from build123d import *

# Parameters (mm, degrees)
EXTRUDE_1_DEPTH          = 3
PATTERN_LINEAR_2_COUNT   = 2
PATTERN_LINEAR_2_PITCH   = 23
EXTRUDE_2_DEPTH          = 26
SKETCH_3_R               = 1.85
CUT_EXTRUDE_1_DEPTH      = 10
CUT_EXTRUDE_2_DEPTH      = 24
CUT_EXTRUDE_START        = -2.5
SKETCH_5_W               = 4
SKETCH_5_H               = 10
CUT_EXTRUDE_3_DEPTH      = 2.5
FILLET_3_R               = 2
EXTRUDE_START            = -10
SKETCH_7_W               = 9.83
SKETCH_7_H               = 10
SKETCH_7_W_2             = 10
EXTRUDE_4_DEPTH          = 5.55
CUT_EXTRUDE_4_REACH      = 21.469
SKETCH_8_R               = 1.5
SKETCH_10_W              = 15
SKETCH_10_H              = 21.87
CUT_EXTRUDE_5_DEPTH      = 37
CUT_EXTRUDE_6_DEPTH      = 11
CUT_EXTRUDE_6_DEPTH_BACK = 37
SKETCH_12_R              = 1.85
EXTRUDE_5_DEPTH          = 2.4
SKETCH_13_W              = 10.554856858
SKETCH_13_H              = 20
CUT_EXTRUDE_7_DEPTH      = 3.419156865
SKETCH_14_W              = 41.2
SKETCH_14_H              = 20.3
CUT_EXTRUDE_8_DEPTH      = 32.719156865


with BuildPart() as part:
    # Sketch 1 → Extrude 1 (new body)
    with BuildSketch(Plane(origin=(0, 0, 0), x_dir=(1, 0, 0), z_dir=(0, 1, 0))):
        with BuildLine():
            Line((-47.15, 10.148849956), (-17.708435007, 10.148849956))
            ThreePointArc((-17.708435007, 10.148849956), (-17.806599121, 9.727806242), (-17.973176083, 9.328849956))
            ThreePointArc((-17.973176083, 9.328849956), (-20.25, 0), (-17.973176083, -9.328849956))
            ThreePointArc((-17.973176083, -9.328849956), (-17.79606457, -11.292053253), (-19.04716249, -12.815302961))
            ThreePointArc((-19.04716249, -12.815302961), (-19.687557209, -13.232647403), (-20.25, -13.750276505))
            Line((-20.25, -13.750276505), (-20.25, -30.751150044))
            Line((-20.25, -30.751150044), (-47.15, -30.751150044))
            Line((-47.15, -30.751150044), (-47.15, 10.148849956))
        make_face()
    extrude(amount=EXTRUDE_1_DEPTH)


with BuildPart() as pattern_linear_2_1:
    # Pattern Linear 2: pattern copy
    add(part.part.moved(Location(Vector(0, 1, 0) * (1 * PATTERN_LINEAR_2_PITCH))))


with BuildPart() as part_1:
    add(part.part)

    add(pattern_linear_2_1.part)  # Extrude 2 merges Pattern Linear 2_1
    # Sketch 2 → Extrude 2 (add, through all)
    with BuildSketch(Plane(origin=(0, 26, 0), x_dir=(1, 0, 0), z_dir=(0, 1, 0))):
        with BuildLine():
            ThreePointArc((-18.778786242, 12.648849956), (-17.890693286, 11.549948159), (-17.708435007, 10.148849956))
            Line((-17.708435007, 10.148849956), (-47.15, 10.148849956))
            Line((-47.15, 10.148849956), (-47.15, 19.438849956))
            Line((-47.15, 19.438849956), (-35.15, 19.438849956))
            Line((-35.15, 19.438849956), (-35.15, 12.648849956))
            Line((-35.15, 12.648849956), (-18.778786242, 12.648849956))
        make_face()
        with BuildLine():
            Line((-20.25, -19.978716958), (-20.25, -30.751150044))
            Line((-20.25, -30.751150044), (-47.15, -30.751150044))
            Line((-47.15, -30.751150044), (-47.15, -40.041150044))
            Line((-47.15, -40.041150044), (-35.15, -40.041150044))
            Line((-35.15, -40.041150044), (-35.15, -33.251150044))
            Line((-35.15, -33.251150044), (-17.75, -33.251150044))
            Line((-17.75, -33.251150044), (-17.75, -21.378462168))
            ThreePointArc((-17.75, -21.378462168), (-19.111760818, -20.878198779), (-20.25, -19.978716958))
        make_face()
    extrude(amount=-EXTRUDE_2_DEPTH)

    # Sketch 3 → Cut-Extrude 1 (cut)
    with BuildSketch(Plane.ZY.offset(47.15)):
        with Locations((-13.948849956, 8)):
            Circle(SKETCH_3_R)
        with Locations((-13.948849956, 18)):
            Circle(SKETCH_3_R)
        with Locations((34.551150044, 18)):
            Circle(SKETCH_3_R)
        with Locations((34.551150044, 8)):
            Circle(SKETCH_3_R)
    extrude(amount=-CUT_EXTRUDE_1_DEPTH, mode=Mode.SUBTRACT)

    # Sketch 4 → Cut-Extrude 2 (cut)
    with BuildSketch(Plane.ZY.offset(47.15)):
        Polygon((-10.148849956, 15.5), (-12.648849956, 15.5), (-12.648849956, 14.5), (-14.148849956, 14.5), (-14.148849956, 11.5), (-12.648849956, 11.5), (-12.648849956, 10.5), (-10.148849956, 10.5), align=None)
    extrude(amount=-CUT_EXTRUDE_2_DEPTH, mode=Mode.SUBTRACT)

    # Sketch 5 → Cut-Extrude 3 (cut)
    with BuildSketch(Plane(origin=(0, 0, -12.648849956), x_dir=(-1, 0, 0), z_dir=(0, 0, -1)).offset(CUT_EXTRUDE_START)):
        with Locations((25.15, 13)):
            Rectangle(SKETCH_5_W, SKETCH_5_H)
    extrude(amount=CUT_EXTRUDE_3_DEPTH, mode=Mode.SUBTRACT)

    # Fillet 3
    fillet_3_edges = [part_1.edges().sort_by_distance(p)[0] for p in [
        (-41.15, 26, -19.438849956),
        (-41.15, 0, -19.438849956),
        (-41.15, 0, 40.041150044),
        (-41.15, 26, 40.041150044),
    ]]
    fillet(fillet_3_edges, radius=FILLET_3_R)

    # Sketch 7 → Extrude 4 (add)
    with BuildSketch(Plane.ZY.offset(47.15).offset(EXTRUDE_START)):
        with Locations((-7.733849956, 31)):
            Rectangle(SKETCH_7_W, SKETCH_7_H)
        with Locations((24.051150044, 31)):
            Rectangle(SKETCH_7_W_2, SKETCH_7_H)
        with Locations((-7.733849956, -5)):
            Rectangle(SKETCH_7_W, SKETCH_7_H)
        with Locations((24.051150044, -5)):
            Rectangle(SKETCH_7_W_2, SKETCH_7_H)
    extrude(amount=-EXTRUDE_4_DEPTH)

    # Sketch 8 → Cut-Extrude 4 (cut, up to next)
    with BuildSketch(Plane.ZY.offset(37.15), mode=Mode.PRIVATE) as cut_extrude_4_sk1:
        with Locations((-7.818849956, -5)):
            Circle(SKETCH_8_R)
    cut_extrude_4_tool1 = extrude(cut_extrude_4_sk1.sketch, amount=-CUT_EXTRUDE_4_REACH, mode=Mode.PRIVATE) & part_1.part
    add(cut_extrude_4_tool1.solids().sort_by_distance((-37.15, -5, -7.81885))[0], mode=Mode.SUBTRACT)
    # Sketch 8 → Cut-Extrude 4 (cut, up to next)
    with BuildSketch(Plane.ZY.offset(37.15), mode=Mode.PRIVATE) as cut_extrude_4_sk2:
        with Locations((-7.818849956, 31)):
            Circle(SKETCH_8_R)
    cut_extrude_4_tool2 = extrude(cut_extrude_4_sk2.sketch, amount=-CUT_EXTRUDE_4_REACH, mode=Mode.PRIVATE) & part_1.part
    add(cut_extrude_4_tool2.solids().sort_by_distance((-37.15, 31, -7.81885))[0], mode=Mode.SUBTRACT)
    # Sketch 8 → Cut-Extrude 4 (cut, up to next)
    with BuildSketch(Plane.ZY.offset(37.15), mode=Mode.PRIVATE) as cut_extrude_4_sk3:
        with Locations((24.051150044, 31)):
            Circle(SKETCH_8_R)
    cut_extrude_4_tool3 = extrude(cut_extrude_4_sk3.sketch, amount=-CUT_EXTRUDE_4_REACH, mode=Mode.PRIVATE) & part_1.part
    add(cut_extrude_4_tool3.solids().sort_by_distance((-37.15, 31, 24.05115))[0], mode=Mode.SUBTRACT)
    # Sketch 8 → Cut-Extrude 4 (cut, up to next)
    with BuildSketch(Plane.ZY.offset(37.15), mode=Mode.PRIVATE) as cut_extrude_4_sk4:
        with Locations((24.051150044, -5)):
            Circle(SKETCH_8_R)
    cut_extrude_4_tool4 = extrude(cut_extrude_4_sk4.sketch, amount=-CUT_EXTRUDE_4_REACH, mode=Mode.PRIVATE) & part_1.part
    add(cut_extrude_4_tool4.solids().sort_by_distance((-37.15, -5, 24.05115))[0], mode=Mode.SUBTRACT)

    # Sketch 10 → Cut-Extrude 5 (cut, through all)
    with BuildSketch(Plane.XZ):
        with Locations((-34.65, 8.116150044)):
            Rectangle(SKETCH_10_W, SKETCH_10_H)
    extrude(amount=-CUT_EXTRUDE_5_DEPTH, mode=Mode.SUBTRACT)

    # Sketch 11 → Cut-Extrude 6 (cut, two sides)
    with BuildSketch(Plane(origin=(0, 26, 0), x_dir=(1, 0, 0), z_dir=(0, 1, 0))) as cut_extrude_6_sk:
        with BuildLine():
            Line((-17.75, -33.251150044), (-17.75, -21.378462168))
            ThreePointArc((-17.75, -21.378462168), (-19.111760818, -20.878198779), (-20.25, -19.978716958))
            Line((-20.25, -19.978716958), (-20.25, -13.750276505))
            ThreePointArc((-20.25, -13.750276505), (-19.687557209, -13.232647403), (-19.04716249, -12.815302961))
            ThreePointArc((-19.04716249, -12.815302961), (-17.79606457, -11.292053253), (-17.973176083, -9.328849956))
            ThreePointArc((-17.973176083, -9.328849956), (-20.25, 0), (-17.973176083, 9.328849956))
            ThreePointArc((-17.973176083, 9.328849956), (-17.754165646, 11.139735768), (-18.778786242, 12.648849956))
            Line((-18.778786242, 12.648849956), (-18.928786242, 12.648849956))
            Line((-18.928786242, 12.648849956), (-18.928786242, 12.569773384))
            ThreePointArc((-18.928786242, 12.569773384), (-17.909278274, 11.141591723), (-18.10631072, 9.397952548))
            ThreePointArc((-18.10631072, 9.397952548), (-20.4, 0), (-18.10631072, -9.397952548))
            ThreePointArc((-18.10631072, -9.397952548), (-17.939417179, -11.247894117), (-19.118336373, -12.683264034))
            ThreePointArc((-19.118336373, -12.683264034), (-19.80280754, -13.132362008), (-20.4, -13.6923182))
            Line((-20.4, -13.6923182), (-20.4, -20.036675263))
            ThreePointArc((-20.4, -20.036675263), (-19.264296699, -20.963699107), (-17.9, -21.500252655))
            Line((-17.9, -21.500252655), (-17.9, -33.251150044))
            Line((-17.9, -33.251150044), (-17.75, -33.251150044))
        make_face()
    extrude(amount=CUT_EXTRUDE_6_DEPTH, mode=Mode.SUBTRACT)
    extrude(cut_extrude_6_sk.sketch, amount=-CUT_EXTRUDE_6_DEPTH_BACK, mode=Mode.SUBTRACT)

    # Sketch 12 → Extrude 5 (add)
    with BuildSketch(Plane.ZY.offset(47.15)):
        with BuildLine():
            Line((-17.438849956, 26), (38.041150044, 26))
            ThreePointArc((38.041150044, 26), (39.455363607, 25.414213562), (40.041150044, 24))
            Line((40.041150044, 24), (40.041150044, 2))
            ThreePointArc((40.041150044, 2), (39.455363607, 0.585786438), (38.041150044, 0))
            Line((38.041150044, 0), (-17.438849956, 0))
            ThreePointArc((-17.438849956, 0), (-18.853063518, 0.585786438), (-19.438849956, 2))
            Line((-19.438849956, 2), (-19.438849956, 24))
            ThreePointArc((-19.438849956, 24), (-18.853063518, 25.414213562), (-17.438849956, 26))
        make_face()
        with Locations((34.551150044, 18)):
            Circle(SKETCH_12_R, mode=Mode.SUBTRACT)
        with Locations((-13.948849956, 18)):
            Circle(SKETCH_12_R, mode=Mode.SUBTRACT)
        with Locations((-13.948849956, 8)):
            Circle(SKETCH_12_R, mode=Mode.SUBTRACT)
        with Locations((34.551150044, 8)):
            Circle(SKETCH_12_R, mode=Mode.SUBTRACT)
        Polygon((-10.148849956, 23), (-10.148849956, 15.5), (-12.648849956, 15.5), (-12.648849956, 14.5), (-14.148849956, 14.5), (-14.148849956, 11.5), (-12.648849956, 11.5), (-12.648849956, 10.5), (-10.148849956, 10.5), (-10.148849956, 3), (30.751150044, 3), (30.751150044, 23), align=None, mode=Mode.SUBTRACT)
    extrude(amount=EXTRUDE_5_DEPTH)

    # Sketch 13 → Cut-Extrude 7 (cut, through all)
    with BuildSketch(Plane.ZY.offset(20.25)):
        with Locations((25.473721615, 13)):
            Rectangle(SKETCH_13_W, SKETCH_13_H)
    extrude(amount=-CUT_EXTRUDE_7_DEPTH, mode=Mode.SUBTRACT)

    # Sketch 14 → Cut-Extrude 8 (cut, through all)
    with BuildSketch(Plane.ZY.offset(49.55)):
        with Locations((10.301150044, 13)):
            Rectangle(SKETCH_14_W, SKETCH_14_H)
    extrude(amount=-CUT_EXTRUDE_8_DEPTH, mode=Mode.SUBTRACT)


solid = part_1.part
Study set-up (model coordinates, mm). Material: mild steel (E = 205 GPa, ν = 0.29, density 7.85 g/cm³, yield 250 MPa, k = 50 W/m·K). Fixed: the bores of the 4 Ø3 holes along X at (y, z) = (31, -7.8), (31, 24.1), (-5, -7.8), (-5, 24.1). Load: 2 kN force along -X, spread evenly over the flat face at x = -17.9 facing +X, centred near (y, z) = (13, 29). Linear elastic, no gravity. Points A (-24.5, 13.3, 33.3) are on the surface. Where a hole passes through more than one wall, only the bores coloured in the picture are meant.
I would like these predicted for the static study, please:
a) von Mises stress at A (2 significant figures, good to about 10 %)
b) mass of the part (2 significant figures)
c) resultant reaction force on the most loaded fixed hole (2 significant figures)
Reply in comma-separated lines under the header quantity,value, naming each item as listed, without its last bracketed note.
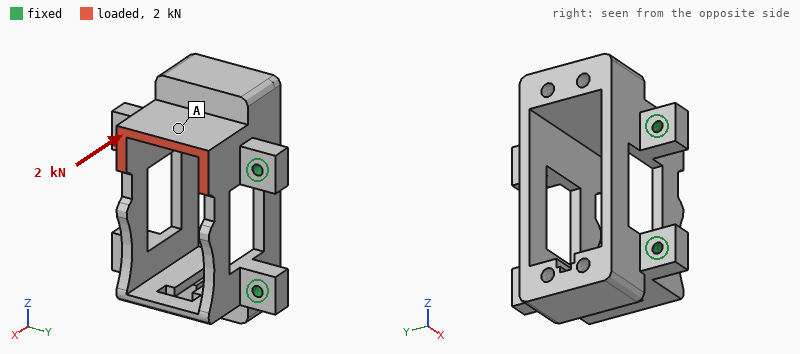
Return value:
quantity,value
von Mises stress at A,11 MPa
mass of the part,120 g
resultant reaction force on the most loaded fixed hole,1.1 kN
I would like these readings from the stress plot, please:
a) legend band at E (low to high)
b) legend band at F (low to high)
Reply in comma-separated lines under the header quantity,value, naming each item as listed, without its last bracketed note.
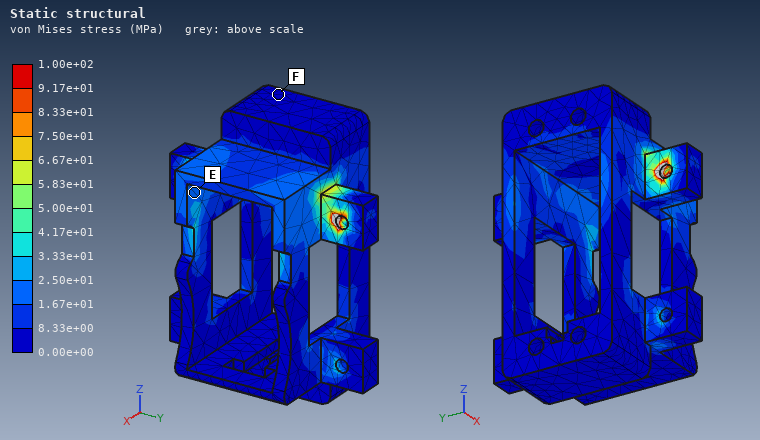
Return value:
quantity,value
legend band at E,1.67e+01 to 2.50e+01 MPa
legend band at F,0.00e+00 to 8.33e+00 MPa
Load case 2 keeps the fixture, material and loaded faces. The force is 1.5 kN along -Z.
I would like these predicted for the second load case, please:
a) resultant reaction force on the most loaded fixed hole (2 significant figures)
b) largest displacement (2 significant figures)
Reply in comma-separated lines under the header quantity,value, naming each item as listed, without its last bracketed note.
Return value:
quantity,value
resultant reaction force on the most loaded fixed hole,600 N
largest displacement,42 µm
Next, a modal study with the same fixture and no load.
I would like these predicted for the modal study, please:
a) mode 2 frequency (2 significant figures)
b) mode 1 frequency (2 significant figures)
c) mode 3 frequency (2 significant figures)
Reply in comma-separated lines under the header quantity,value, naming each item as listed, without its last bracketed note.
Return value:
quantity,value
mode 2 frequency,9300 Hz
mode 1 frequency,8100 Hz
mode 3 frequency,9900 Hz
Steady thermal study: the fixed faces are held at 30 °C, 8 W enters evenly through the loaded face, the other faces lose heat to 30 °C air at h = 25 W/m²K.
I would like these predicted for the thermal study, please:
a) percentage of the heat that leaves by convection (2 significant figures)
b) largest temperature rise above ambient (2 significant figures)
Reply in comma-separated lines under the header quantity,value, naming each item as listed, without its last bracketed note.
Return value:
quantity,value
percentage of the heat that leaves by convection,19 %
largest temperature rise above ambient,28 K
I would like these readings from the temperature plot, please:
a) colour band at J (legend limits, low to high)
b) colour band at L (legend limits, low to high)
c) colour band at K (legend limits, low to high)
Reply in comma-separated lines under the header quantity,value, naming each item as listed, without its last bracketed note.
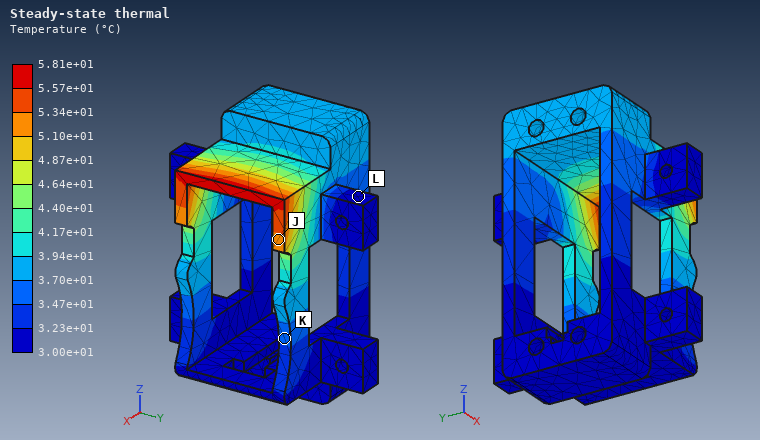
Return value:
quantity,value
colour band at J,5.10e+01 to 5.34e+01 °C
colour band at L,3.00e+01 to 3.23e+01 °C
colour band at K,3.47e+01 to 3.70e+01 °C
